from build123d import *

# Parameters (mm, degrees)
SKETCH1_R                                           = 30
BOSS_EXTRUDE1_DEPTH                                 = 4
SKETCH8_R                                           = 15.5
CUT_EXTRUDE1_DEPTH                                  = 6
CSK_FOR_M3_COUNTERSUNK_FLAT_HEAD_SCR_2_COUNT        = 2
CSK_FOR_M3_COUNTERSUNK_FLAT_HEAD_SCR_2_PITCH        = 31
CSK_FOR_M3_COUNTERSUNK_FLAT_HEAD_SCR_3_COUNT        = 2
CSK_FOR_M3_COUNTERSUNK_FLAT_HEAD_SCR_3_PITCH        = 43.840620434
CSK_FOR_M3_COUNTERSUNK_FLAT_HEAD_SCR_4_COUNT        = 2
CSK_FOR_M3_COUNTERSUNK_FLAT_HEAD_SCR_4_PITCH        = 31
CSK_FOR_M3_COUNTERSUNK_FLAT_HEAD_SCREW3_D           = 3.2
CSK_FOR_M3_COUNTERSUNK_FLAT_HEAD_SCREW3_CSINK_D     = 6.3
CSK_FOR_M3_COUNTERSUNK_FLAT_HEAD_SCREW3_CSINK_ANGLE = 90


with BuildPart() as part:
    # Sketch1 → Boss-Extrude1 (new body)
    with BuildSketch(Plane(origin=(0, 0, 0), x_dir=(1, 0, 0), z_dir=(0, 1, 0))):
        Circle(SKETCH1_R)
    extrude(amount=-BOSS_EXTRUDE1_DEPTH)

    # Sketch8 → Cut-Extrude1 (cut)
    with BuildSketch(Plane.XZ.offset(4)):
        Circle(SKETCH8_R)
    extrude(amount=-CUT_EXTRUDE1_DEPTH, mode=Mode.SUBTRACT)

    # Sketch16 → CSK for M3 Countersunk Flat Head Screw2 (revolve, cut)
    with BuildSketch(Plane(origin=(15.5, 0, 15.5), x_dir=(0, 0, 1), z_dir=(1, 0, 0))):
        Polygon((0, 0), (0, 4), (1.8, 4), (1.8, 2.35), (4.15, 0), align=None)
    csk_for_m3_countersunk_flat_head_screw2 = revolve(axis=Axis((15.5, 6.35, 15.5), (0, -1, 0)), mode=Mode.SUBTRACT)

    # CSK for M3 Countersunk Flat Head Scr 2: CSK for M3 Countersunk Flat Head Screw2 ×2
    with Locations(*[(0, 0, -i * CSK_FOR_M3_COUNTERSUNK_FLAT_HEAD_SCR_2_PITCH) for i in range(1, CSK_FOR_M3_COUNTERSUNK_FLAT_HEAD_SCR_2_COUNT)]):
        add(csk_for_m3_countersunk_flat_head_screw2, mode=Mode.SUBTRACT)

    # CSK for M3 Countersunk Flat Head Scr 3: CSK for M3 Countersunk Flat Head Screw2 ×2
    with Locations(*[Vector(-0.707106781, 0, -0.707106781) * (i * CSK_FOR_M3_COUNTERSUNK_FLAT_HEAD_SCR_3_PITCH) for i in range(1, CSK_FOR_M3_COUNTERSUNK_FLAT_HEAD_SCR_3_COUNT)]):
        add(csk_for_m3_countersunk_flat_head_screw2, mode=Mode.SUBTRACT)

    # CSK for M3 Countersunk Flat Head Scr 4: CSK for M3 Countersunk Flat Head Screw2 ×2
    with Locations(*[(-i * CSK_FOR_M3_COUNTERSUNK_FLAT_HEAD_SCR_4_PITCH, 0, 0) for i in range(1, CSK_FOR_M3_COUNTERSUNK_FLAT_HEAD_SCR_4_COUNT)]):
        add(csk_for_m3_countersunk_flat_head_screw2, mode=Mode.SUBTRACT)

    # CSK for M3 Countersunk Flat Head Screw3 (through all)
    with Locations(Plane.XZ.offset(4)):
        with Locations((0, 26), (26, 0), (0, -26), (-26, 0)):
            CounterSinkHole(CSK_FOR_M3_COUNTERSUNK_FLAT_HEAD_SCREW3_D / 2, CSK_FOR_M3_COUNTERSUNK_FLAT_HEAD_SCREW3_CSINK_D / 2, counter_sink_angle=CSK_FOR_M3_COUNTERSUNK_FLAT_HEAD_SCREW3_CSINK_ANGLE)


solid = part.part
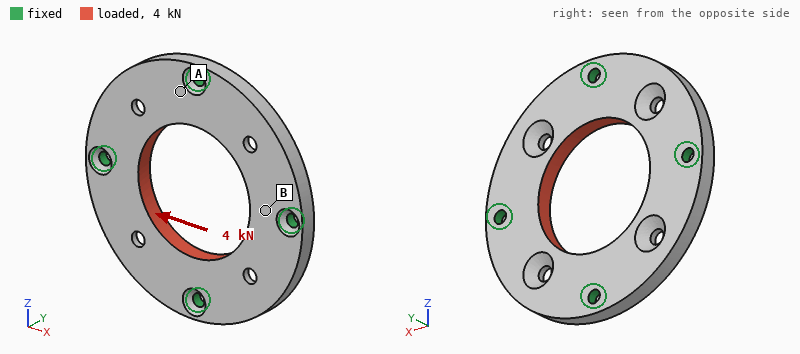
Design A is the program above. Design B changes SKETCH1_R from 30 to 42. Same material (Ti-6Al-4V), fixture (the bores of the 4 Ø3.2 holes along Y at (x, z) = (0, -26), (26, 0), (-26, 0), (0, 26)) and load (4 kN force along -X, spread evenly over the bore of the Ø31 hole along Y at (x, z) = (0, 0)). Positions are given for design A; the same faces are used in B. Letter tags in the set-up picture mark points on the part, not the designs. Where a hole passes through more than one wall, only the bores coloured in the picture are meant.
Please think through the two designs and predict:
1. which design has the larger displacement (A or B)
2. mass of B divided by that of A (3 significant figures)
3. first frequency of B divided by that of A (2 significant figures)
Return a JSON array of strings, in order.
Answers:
["A", "2.40", "0.46"]
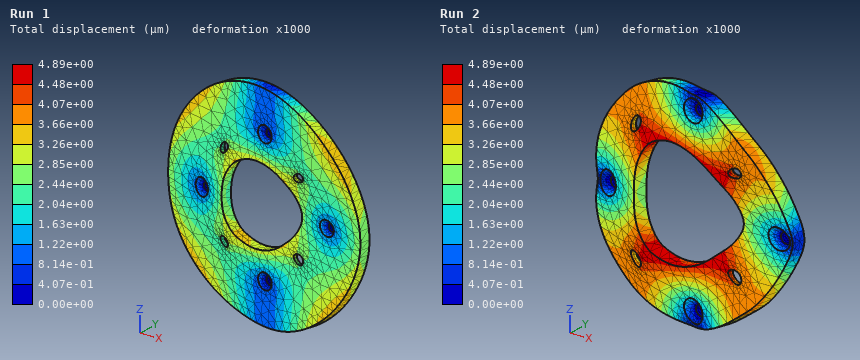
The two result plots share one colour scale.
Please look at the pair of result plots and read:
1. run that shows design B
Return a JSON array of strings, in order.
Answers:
["Run 1"]
